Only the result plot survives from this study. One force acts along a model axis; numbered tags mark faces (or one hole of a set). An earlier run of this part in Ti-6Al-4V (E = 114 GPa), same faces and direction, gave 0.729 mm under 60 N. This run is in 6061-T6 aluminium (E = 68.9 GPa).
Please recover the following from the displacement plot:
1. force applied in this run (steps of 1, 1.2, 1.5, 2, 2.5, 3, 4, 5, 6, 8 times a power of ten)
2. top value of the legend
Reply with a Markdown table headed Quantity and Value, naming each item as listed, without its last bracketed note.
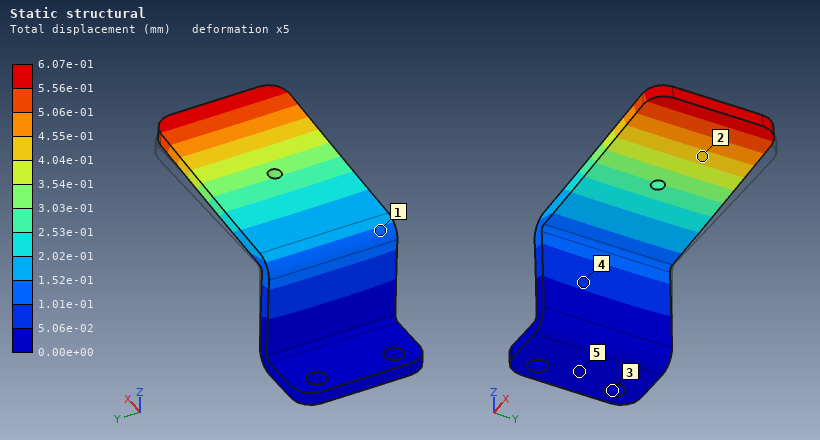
| Quantity | Value |
|---|---|
| force applied in this run | 30 N |
| top value of the legend | 6.07e-01 mm |
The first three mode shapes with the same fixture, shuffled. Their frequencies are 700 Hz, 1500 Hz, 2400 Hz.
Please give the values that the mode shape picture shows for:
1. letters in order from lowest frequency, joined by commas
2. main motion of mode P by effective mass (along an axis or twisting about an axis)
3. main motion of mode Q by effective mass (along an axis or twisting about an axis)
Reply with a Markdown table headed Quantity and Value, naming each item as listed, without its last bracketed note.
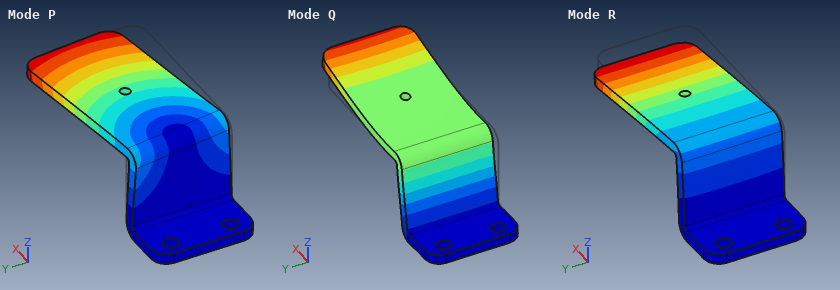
| Quantity | Value |
|---|---|
| letters in order from lowest frequency, joined by commas | R, P, Q |
| main motion of mode P by effective mass | along Y |
| main motion of mode Q by effective mass | along X |
